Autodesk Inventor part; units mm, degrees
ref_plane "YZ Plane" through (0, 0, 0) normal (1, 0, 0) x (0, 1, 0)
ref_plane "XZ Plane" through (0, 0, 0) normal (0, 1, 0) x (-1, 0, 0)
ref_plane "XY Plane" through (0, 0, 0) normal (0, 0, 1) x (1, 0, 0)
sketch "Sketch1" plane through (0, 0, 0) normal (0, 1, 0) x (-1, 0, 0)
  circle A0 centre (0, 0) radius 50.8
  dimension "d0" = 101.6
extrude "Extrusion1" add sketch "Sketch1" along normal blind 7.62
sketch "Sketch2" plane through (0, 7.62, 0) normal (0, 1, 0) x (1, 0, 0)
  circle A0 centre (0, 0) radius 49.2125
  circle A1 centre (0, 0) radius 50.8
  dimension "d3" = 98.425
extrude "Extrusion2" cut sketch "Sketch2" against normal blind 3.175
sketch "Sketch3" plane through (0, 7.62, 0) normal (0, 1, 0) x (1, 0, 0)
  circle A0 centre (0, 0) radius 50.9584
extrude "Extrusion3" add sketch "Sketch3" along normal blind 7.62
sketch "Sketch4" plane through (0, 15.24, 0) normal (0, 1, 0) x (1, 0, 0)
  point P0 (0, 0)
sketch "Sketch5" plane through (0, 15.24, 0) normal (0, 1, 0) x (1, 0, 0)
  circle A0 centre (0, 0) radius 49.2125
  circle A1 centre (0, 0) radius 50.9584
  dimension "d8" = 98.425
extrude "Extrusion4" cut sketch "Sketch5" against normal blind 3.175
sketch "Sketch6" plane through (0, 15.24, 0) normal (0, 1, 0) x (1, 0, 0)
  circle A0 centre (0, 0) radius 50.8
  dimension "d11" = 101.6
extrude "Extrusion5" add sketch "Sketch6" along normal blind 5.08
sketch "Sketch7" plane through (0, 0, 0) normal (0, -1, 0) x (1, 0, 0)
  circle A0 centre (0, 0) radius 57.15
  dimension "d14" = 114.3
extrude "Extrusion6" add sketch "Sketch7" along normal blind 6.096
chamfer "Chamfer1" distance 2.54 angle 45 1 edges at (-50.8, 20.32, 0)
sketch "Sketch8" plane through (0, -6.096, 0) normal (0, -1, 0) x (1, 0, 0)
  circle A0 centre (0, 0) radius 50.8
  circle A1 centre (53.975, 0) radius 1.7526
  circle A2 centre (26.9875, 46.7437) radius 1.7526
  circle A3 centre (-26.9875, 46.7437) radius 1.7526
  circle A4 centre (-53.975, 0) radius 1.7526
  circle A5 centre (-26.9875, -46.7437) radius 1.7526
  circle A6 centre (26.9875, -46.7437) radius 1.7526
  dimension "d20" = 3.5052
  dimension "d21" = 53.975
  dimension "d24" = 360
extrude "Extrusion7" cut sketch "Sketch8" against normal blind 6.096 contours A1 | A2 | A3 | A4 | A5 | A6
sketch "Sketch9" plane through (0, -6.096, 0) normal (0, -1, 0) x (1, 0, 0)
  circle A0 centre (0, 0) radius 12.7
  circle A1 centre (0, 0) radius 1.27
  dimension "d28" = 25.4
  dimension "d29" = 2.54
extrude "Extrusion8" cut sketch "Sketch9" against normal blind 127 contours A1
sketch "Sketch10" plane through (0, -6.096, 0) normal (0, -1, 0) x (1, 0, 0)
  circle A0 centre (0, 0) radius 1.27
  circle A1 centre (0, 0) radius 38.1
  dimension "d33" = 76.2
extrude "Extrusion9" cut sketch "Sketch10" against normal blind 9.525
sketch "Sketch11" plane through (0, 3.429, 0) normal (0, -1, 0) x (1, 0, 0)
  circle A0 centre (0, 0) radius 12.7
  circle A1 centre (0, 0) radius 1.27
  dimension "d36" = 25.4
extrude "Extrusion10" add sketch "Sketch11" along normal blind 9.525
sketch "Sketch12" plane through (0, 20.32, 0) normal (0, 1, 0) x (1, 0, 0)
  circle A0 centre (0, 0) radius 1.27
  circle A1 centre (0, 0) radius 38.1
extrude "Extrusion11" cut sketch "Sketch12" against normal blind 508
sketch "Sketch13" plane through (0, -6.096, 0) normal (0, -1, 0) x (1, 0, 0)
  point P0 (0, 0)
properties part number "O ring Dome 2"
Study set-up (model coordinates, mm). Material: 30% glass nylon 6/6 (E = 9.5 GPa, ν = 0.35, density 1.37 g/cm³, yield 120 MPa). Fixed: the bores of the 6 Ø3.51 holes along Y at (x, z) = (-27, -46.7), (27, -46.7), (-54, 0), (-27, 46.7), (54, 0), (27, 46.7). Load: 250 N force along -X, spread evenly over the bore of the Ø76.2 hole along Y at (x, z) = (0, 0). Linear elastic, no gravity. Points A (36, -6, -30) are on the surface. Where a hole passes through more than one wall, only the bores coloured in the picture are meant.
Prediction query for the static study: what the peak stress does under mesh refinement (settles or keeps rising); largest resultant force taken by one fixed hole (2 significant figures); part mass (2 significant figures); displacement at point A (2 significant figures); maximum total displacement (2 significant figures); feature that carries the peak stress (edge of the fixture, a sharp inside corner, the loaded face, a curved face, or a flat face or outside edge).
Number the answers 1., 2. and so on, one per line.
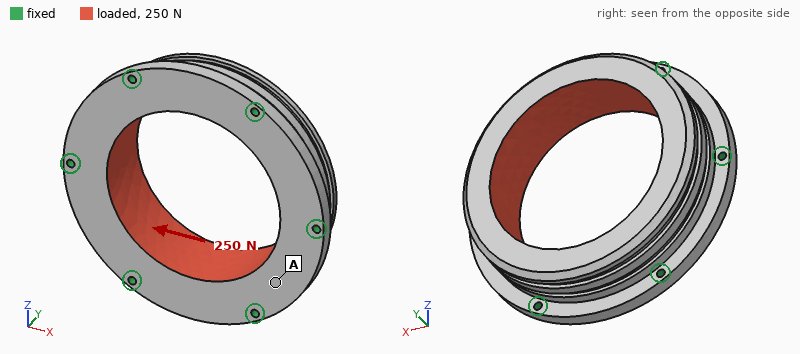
1. keeps rising
2. 44 N
3. 140 g
4. 0.75 µm
5. 1.8 µm
6. edge of the fixture
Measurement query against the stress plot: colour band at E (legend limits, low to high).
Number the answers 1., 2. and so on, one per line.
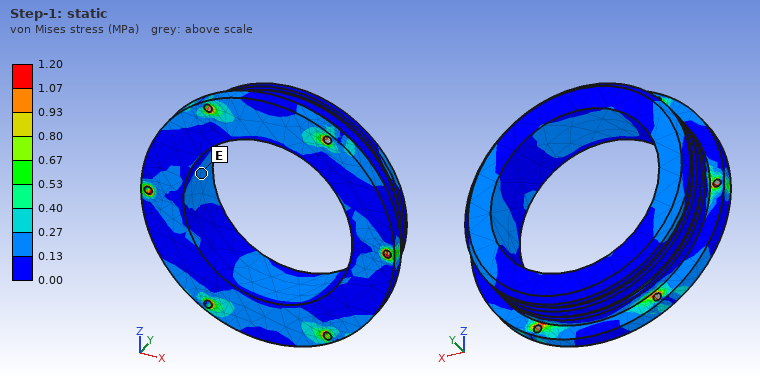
1. 0.13 to 0.27 MPa
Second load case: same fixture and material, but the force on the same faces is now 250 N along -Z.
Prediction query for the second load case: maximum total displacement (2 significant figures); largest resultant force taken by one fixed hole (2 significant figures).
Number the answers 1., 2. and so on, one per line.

1. 2.0 µm
2. 44 N
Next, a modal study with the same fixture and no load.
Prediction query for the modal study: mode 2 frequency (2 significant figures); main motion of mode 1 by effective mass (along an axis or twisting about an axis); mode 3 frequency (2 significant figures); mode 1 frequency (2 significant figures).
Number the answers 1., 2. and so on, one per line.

1. 5600 Hz
2. along Y
3. 5600 Hz
4. 5300 Hz
